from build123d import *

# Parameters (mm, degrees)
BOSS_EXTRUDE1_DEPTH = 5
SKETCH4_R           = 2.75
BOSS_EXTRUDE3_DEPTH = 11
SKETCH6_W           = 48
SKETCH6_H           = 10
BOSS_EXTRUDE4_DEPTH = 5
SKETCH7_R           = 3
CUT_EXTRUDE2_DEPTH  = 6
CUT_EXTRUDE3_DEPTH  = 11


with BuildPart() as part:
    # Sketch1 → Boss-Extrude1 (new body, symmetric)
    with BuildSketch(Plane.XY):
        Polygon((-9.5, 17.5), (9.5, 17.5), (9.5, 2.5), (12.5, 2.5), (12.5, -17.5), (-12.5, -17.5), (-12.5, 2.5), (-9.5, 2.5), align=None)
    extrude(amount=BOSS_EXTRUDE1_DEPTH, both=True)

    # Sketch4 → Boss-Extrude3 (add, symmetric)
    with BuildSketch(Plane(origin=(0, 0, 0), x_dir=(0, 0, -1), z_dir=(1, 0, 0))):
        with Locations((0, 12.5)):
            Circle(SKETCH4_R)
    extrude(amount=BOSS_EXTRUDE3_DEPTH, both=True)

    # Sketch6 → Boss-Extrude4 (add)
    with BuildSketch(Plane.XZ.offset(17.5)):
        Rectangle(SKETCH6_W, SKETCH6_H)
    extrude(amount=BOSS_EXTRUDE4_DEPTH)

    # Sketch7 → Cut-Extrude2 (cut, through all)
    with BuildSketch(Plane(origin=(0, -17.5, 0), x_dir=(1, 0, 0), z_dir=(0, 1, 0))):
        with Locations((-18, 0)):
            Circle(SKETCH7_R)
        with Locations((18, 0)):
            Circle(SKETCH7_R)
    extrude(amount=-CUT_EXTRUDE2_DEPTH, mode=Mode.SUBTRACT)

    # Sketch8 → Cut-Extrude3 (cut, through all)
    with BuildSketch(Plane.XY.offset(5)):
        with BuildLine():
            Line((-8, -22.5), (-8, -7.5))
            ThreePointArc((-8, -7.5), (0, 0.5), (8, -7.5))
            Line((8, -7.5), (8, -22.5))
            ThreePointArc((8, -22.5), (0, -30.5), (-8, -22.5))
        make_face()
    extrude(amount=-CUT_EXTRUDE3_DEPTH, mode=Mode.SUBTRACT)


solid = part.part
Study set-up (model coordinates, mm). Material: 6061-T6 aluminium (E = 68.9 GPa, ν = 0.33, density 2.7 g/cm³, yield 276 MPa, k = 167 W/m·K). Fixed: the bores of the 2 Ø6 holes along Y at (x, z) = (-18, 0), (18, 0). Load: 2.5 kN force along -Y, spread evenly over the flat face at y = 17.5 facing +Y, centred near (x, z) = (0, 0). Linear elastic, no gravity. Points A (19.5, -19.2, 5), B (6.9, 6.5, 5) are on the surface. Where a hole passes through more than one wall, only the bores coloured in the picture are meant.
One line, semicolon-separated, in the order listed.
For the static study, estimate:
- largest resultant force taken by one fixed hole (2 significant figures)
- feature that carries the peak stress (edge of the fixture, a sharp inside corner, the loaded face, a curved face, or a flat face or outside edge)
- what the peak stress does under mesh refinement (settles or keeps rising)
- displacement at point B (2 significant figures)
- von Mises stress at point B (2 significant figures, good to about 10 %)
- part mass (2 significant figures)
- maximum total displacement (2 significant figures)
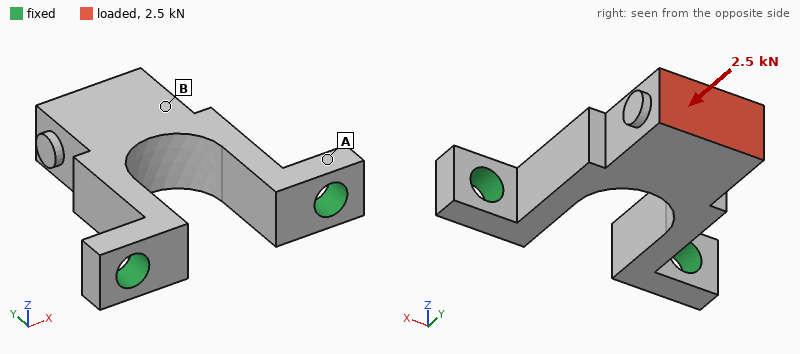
1.3 kN; edge of the fixture; keeps rising; 19 µm; 19 MPa; 18 g; 22 µm
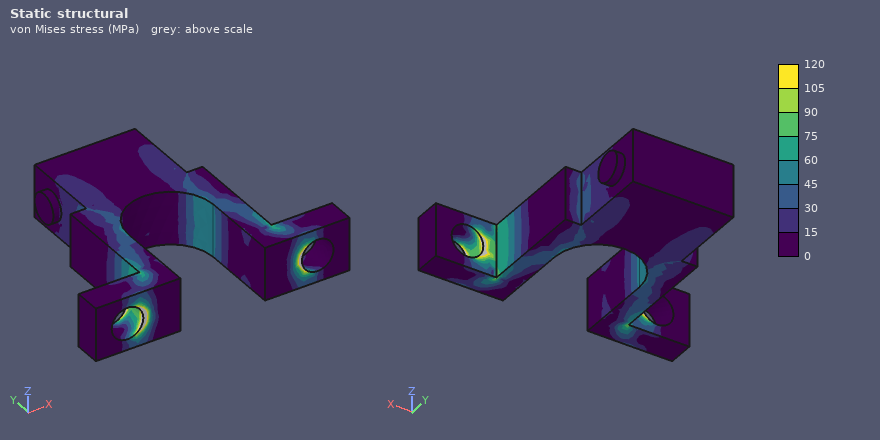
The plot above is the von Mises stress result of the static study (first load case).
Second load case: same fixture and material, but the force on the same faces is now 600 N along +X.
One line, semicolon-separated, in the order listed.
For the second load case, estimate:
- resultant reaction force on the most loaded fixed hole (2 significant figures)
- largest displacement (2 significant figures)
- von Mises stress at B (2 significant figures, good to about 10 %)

860 N; 49 µm; 8.5 MPa
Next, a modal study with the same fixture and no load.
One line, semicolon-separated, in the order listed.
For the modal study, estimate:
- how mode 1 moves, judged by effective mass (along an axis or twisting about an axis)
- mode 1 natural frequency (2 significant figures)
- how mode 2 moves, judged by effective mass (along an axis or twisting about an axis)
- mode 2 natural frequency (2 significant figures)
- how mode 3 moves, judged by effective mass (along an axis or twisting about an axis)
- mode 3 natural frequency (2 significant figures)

along Z; 2600 Hz; along X; 5800 Hz; twisting about Y; 9600 Hz
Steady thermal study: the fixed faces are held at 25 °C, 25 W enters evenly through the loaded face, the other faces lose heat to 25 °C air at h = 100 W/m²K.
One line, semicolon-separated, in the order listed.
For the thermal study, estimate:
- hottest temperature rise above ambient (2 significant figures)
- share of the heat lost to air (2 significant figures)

42 K; 26 %
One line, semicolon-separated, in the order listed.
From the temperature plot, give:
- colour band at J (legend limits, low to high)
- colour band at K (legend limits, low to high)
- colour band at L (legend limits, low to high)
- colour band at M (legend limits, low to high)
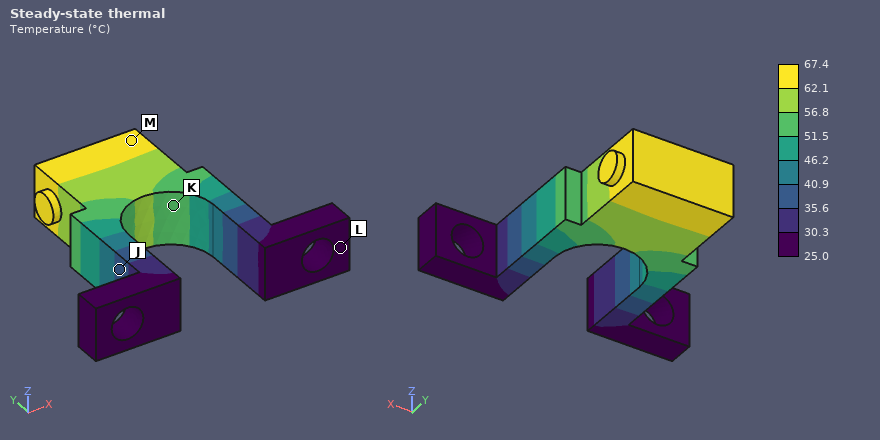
35.6 to 40.9 °C; 51.5 to 56.8 °C; 25.0 to 30.3 °C; 62.1 to 67.4 °C
